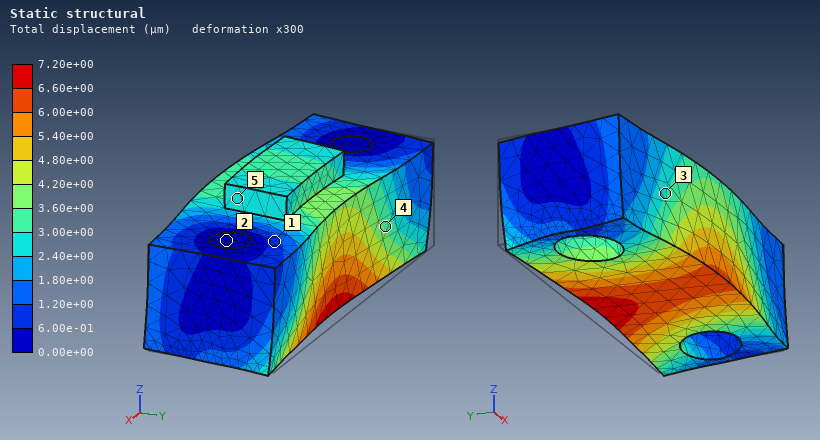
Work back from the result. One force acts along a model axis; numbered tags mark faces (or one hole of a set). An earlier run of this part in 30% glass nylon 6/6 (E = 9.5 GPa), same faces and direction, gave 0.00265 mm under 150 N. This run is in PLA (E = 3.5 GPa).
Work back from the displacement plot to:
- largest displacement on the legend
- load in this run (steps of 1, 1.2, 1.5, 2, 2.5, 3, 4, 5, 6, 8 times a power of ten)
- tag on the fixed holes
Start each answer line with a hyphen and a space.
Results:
- 7.20e+00 µm
- 150 N
- 2
